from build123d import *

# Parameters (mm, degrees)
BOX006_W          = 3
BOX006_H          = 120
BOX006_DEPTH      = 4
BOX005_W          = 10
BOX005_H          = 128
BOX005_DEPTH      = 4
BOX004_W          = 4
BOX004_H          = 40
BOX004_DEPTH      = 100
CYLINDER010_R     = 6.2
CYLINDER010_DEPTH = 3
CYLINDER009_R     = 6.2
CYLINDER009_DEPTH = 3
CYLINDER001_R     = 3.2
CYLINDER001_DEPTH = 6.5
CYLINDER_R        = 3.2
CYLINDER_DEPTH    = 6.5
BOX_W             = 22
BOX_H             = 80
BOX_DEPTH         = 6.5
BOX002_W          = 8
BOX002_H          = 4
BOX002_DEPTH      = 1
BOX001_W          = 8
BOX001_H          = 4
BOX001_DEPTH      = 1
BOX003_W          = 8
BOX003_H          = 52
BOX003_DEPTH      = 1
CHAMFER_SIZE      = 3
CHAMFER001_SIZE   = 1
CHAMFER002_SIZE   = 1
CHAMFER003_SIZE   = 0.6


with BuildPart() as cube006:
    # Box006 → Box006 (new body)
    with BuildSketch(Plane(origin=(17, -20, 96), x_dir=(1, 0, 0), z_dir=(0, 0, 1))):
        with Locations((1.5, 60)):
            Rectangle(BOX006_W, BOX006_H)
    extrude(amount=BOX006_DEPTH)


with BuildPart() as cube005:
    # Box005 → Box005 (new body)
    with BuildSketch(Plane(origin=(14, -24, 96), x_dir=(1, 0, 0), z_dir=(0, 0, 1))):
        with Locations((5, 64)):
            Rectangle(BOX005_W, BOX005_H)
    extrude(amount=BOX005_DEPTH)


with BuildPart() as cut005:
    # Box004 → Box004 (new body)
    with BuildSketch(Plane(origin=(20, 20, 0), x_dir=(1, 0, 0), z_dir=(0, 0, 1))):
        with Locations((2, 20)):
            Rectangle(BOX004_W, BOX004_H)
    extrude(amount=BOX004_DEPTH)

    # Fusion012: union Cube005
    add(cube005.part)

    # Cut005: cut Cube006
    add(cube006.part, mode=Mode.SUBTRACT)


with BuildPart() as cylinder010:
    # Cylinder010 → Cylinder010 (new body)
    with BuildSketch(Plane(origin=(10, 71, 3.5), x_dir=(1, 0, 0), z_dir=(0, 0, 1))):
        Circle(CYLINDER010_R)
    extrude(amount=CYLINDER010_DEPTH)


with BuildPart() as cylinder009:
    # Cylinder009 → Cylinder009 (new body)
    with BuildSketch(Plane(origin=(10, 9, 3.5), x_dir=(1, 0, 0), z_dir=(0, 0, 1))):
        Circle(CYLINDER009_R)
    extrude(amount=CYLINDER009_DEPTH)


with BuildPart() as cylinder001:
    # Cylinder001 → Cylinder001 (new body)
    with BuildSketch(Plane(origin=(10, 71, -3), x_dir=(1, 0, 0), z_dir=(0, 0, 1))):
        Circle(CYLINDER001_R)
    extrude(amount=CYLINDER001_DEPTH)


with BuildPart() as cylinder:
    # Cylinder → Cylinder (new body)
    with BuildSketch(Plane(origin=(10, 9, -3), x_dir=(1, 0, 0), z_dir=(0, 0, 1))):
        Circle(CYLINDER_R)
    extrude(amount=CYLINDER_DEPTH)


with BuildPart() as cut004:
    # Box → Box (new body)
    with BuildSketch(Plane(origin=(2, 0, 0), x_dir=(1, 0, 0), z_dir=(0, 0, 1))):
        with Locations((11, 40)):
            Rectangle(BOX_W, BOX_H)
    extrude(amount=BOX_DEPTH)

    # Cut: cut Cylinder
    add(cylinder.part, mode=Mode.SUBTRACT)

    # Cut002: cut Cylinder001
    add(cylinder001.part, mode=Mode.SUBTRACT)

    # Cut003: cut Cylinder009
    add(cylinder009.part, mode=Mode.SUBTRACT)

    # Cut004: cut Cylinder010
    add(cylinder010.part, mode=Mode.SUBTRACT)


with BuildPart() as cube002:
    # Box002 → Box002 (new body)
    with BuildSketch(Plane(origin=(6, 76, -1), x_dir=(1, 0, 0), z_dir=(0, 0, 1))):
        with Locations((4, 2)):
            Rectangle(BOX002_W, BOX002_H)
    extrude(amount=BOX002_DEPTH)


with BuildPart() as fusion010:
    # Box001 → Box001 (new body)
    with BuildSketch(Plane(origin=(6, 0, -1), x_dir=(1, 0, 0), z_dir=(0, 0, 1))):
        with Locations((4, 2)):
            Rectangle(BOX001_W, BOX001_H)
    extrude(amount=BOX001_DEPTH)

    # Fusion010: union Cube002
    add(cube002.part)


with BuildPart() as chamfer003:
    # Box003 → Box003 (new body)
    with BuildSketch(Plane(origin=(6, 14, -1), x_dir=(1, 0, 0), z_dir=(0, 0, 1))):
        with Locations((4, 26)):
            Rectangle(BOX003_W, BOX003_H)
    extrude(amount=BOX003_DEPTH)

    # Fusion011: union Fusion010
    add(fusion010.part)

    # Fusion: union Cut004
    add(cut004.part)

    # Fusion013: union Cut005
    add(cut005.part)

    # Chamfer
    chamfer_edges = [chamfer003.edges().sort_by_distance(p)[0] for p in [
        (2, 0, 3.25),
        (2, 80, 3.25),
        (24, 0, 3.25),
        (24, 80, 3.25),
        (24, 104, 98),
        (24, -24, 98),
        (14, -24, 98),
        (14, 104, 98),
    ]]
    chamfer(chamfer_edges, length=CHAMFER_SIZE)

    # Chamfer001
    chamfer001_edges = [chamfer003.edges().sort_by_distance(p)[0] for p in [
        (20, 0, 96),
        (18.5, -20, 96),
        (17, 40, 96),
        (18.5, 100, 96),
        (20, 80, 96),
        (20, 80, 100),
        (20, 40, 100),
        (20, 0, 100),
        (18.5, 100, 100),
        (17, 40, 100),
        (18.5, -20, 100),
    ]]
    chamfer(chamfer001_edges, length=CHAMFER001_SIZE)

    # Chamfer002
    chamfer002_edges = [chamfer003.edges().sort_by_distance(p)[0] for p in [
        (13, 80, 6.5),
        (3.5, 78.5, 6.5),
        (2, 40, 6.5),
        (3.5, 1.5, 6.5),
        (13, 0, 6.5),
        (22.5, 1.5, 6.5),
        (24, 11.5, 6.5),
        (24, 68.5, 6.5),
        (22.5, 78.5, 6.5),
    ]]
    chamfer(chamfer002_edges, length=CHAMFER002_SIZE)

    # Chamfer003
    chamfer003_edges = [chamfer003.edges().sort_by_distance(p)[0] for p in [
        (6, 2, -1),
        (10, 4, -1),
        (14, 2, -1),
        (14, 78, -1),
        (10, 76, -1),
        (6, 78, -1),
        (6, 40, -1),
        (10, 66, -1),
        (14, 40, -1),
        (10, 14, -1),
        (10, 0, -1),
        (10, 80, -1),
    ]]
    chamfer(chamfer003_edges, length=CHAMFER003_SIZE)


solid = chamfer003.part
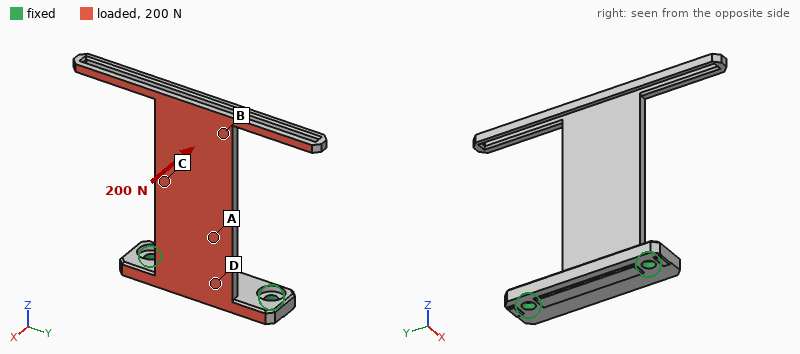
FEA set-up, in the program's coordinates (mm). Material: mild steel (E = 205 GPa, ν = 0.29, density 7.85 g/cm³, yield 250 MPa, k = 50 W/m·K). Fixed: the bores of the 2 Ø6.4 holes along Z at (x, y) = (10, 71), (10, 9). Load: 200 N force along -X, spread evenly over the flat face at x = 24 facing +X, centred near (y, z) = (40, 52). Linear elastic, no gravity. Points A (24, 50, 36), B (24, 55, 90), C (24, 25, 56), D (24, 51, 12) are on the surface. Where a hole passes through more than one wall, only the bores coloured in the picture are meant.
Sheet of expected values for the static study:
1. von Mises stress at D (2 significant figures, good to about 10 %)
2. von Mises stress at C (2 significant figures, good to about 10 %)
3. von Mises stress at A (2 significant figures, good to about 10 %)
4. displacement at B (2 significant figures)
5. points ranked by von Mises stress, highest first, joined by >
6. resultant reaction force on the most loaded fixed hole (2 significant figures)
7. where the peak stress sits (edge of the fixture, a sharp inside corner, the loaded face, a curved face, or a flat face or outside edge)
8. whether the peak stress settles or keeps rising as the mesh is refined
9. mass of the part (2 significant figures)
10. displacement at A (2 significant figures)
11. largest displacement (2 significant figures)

68 MPa
22 MPa
42 MPa
0.52 mm
D > A > C > B
140 N
edge of the fixture
keeps rising
220 g
0.12 mm
0.61 mm
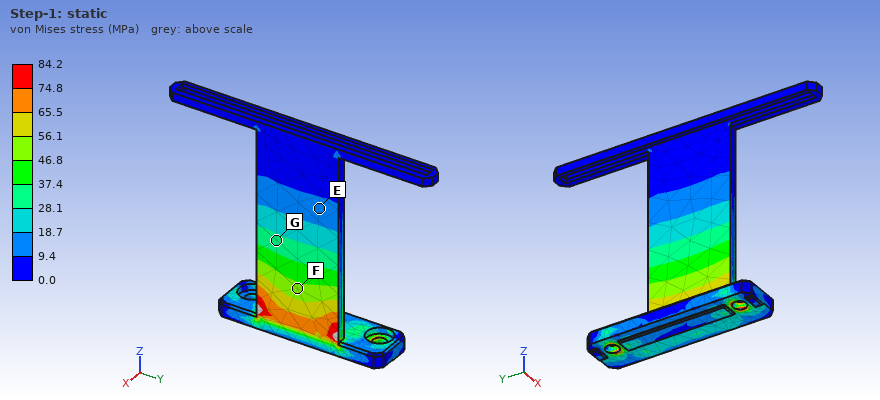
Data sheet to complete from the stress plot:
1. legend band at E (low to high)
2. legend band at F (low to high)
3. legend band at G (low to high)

9.4 to 18.7 MPa
46.8 to 56.1 MPa
28.1 to 37.4 MPa
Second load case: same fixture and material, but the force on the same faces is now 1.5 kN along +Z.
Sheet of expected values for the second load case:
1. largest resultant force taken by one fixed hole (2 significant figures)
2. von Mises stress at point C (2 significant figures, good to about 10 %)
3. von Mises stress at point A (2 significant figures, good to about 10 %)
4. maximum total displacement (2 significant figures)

860 N
17 MPa
24 MPa
0.39 mm
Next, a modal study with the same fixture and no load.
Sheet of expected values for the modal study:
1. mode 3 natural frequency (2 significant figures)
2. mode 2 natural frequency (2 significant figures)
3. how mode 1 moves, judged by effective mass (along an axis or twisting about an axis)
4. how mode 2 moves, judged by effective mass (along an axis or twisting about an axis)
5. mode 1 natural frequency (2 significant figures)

850 Hz
570 Hz
along X
twisting about Z
260 Hz
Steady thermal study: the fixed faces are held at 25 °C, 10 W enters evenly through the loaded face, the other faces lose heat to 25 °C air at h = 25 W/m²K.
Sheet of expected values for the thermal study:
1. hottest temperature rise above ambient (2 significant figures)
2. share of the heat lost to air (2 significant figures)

34 K
47 %
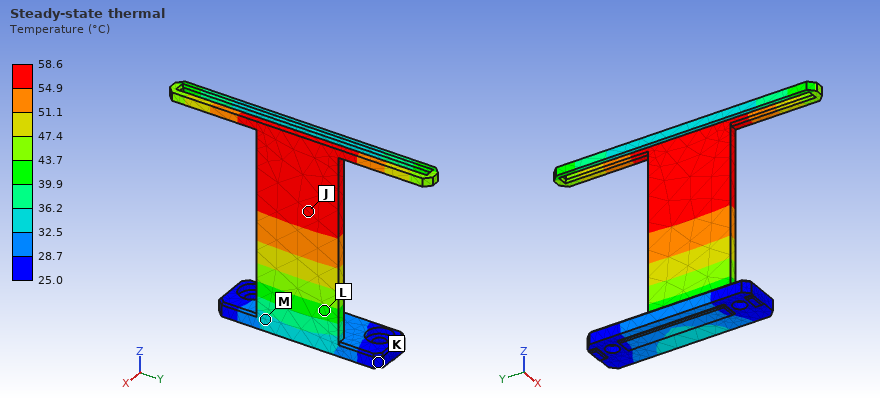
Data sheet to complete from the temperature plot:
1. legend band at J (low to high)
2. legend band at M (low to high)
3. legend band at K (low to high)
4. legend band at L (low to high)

54.9 to 58.6 °C
32.5 to 36.2 °C
25.0 to 28.7 °C
39.9 to 43.7 °C
